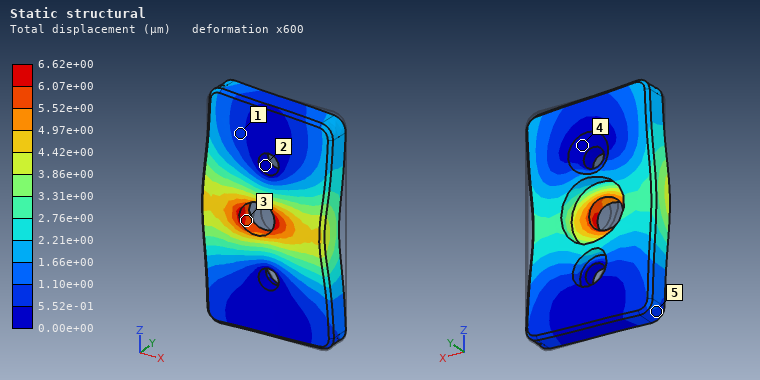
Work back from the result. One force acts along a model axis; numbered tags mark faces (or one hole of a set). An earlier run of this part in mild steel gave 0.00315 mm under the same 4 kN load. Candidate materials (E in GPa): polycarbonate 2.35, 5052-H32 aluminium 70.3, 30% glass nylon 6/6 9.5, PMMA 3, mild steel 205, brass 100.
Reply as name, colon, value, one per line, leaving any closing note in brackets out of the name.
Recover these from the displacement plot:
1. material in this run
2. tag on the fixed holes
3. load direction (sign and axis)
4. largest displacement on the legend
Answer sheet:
material in this run: brass
tag on the fixed holes: 2
load direction: -X
largest displacement on the legend: 6.62e+00 µm
